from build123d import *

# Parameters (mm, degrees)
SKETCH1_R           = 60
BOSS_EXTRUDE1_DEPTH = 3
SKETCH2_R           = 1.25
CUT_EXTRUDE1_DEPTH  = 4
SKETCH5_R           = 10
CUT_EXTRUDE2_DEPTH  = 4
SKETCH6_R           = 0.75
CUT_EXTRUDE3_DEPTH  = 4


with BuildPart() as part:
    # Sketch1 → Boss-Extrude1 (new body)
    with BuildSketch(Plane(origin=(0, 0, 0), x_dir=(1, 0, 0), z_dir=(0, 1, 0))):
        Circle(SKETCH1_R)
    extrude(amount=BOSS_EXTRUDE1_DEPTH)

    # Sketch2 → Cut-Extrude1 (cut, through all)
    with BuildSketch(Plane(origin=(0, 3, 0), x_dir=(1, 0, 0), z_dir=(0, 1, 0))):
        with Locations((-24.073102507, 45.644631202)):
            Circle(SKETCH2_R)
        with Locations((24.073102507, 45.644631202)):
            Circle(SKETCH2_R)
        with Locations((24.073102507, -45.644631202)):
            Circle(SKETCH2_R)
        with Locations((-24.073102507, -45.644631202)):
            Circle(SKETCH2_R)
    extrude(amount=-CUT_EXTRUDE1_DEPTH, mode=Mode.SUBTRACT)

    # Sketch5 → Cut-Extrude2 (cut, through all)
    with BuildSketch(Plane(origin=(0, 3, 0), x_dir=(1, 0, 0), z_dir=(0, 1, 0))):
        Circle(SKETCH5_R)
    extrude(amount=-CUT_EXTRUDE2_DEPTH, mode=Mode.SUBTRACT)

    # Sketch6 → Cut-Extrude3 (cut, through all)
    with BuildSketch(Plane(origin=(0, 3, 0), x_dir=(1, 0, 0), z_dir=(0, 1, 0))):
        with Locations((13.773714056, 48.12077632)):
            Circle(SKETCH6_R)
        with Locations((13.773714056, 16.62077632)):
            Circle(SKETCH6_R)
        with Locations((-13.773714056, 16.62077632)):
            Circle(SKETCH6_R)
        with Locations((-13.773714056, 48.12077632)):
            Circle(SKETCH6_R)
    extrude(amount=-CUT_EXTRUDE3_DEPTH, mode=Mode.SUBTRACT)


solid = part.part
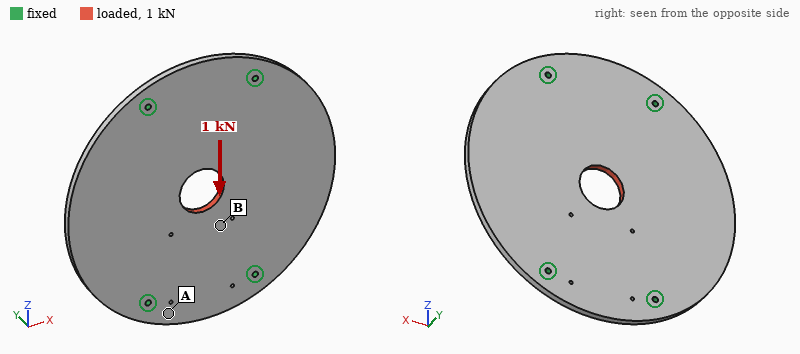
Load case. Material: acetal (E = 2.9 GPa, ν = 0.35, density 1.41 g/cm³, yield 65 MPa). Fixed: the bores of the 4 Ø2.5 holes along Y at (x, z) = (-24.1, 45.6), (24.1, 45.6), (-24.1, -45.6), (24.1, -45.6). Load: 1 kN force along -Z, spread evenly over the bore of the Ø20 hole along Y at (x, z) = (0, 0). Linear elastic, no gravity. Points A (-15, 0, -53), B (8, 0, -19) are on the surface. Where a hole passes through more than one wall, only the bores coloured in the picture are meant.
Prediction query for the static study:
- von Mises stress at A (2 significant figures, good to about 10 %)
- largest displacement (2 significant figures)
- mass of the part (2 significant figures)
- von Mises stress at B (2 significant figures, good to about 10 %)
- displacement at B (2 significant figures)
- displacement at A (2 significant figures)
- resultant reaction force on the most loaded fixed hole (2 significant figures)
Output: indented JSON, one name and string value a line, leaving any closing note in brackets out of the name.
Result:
{
  "von Mises stress at A": "1.7 MPa",
  "largest displacement": "73 µm",
  "mass of the part": "46 g",
  "von Mises stress at B": "4.0 MPa",
  "displacement at B": "52 µm",
  "displacement at A": "23 µm",
  "resultant reaction force on the most loaded fixed hole": "250 N"
}
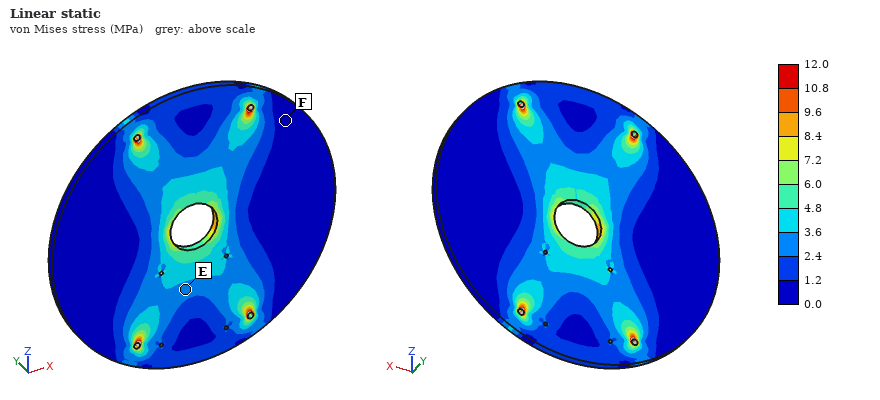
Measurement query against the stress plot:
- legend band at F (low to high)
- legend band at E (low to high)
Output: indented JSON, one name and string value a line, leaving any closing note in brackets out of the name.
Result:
{
  "legend band at F": "0.0 to 1.2 MPa",
  "legend band at E": "2.4 to 3.6 MPa"
}
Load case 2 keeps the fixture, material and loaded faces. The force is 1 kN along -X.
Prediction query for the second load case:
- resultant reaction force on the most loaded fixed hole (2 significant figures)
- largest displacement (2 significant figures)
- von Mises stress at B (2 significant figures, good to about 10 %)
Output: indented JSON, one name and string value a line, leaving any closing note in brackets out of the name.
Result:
{
  "resultant reaction force on the most loaded fixed hole": "260 N",
  "largest displacement": "0.11 mm",
  "von Mises stress at B": "3.9 MPa"
}
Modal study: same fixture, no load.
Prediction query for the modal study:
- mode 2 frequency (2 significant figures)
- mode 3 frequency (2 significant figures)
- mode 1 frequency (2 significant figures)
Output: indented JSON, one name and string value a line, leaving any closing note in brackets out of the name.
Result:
{
  "mode 2 frequency": "350 Hz",
  "mode 3 frequency": "580 Hz",
  "mode 1 frequency": "350 Hz"
}
